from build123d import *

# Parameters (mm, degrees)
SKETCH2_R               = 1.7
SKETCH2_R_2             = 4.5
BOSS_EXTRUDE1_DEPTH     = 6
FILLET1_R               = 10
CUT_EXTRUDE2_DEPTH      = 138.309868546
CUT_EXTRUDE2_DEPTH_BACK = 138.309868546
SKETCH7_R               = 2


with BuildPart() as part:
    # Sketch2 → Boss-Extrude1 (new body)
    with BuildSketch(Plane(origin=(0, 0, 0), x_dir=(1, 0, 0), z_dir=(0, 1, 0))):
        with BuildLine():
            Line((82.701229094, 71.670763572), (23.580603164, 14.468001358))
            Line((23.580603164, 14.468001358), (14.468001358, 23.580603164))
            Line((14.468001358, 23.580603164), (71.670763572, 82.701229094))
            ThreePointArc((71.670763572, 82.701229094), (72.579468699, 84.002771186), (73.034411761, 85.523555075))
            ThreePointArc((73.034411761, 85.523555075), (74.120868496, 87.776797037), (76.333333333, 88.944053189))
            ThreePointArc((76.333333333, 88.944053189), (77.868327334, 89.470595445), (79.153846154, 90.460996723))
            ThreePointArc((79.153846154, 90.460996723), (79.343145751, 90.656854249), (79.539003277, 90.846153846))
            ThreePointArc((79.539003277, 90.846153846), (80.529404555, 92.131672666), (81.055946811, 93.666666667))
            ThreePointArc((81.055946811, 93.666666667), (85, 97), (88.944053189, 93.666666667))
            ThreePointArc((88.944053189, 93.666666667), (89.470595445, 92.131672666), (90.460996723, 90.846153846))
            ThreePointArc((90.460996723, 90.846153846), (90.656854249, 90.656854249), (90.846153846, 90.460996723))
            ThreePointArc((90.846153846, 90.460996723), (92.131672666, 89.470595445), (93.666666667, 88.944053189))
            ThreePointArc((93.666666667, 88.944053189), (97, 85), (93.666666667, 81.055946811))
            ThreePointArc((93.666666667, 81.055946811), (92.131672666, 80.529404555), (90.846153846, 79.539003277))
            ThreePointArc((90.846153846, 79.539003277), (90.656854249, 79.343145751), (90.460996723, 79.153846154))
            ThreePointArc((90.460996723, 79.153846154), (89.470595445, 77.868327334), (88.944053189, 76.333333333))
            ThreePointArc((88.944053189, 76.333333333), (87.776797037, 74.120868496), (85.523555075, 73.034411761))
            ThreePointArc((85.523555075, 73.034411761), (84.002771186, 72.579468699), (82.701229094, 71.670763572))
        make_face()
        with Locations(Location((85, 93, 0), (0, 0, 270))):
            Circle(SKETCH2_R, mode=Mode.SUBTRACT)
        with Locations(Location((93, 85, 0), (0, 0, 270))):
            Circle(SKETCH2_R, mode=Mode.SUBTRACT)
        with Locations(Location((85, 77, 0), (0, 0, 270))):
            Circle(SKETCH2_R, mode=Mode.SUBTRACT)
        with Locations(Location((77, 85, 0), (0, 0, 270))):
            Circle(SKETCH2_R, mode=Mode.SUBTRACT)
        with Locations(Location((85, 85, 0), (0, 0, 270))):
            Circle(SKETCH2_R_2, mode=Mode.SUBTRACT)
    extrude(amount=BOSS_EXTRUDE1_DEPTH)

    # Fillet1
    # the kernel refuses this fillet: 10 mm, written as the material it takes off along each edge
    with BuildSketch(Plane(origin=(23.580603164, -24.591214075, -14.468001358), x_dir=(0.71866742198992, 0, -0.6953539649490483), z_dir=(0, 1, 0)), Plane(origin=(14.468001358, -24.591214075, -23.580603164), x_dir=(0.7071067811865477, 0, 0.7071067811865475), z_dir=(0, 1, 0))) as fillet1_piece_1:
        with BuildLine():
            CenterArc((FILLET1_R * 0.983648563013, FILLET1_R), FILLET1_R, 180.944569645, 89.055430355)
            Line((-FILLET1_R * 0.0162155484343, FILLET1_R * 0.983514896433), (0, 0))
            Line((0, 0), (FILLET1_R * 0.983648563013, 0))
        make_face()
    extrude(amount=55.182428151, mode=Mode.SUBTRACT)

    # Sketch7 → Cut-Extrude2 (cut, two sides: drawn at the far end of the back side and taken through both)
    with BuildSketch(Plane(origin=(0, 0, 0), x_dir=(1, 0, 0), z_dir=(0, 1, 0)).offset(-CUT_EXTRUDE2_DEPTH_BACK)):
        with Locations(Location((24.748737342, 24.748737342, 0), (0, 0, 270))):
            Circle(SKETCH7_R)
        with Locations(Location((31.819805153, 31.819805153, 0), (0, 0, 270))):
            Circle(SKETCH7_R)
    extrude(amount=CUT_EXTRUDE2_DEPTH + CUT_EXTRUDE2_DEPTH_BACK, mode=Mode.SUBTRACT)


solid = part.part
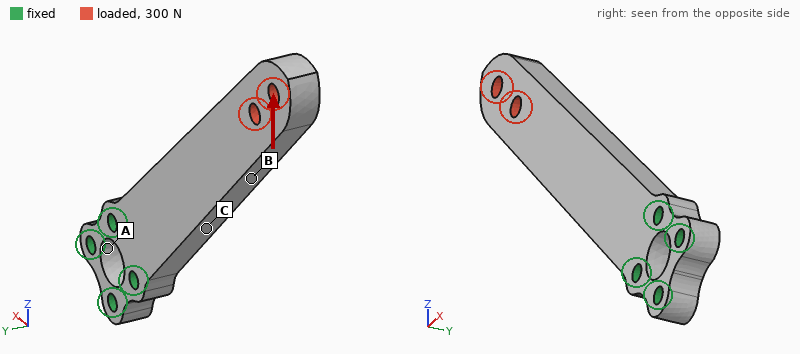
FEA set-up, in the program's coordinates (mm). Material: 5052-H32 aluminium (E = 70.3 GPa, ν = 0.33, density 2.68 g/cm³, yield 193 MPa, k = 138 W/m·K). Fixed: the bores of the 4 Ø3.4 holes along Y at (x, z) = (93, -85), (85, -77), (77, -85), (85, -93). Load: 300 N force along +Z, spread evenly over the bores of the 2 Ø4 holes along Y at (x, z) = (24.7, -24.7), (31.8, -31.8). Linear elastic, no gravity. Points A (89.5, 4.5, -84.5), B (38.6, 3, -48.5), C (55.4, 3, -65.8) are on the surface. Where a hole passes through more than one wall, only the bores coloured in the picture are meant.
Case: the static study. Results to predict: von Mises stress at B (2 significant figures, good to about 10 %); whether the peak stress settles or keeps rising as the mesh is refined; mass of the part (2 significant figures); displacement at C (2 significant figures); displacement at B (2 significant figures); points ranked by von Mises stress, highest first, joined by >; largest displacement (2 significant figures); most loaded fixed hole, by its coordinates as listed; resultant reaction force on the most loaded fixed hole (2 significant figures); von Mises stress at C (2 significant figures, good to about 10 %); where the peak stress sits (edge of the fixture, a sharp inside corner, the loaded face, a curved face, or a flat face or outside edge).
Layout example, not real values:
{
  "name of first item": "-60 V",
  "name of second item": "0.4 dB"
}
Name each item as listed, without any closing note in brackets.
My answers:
{
  "von Mises stress at B": "26 MPa",
  "whether the peak stress settles or keeps rising as the mesh is refined": "keeps rising",
  "mass of the part": "22 g",
  "displacement at C": "0.047 mm",
  "displacement at B": "0.13 mm",
  "points ranked by von Mises stress, highest first, joined by >": "C > B > A",
  "largest displacement": "0.30 mm",
  "most loaded fixed hole, by its coordinates as listed": "(77, -85)",
  "resultant reaction force on the most loaded fixed hole": "1.4 kN",
  "von Mises stress at C": "46 MPa",
  "where the peak stress sits": "edge of the fixture"
}
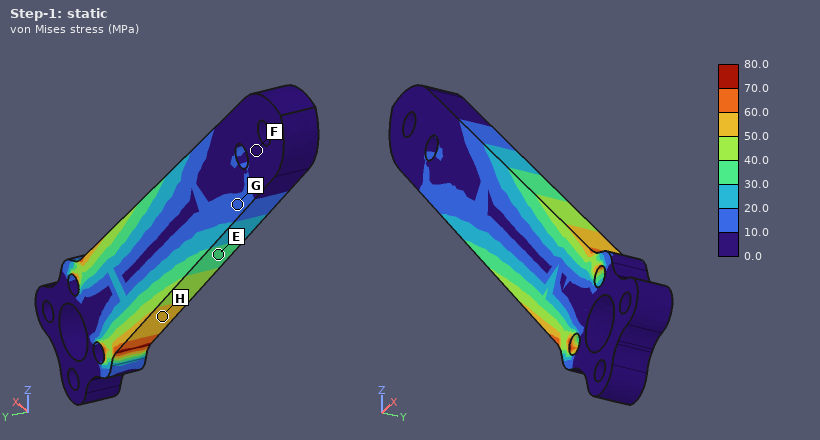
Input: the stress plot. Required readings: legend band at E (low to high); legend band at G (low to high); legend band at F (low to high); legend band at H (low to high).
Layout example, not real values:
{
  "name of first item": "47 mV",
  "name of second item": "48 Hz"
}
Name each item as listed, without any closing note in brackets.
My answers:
{
  "legend band at E": "30.0 to 40.0 MPa",
  "legend band at G": "10.0 to 20.0 MPa",
  "legend band at F": "0.0 to 10.0 MPa",
  "legend band at H": "50.0 to 60.0 MPa"
}
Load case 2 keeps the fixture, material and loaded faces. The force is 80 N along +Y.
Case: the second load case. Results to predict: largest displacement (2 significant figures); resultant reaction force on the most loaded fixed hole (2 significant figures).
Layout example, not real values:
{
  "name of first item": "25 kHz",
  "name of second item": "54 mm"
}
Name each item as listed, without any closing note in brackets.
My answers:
{
  "largest displacement": "0.71 mm",
  "resultant reaction force on the most loaded fixed hole": "50 N"
}
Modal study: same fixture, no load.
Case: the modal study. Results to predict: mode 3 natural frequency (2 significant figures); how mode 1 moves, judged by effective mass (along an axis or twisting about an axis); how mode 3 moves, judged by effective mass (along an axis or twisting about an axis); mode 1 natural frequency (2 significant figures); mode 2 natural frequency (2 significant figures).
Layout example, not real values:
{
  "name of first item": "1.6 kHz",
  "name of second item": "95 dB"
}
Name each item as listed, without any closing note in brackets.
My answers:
{
  "mode 3 natural frequency": "4400 Hz",
  "how mode 1 moves, judged by effective mass": "along Y",
  "how mode 3 moves, judged by effective mass": "along Y",
  "mode 1 natural frequency": "770 Hz",
  "mode 2 natural frequency": "1900 Hz"
}
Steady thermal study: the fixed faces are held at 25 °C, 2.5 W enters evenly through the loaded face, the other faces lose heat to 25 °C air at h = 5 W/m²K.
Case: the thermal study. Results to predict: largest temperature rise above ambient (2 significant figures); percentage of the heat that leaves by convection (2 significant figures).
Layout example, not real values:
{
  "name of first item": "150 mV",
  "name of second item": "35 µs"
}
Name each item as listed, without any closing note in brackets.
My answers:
{
  "largest temperature rise above ambient": "15 K",
  "percentage of the heat that leaves by convection": "5.4 %"
}
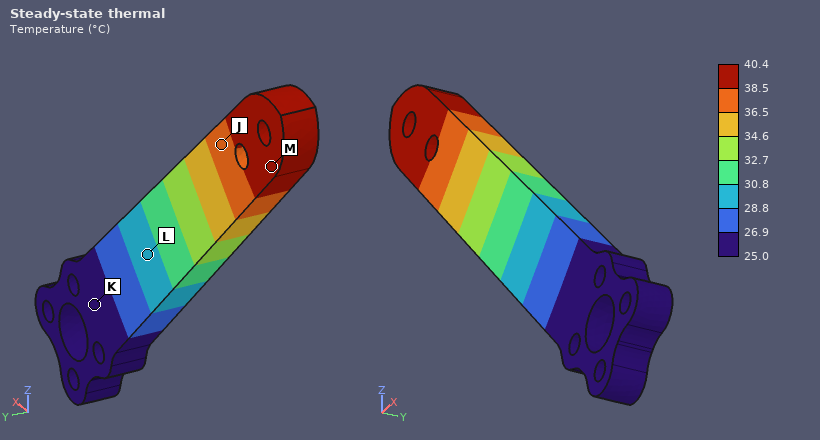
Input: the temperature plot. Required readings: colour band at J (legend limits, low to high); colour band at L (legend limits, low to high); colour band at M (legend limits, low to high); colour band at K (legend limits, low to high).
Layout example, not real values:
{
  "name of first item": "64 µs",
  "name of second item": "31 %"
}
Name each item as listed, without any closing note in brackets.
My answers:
{
  "colour band at J": "36.5 to 38.5 °C",
  "colour band at L": "28.8 to 30.8 °C",
  "colour band at M": "38.5 to 40.4 °C",
  "colour band at K": "25.0 to 26.9 °C"
}
